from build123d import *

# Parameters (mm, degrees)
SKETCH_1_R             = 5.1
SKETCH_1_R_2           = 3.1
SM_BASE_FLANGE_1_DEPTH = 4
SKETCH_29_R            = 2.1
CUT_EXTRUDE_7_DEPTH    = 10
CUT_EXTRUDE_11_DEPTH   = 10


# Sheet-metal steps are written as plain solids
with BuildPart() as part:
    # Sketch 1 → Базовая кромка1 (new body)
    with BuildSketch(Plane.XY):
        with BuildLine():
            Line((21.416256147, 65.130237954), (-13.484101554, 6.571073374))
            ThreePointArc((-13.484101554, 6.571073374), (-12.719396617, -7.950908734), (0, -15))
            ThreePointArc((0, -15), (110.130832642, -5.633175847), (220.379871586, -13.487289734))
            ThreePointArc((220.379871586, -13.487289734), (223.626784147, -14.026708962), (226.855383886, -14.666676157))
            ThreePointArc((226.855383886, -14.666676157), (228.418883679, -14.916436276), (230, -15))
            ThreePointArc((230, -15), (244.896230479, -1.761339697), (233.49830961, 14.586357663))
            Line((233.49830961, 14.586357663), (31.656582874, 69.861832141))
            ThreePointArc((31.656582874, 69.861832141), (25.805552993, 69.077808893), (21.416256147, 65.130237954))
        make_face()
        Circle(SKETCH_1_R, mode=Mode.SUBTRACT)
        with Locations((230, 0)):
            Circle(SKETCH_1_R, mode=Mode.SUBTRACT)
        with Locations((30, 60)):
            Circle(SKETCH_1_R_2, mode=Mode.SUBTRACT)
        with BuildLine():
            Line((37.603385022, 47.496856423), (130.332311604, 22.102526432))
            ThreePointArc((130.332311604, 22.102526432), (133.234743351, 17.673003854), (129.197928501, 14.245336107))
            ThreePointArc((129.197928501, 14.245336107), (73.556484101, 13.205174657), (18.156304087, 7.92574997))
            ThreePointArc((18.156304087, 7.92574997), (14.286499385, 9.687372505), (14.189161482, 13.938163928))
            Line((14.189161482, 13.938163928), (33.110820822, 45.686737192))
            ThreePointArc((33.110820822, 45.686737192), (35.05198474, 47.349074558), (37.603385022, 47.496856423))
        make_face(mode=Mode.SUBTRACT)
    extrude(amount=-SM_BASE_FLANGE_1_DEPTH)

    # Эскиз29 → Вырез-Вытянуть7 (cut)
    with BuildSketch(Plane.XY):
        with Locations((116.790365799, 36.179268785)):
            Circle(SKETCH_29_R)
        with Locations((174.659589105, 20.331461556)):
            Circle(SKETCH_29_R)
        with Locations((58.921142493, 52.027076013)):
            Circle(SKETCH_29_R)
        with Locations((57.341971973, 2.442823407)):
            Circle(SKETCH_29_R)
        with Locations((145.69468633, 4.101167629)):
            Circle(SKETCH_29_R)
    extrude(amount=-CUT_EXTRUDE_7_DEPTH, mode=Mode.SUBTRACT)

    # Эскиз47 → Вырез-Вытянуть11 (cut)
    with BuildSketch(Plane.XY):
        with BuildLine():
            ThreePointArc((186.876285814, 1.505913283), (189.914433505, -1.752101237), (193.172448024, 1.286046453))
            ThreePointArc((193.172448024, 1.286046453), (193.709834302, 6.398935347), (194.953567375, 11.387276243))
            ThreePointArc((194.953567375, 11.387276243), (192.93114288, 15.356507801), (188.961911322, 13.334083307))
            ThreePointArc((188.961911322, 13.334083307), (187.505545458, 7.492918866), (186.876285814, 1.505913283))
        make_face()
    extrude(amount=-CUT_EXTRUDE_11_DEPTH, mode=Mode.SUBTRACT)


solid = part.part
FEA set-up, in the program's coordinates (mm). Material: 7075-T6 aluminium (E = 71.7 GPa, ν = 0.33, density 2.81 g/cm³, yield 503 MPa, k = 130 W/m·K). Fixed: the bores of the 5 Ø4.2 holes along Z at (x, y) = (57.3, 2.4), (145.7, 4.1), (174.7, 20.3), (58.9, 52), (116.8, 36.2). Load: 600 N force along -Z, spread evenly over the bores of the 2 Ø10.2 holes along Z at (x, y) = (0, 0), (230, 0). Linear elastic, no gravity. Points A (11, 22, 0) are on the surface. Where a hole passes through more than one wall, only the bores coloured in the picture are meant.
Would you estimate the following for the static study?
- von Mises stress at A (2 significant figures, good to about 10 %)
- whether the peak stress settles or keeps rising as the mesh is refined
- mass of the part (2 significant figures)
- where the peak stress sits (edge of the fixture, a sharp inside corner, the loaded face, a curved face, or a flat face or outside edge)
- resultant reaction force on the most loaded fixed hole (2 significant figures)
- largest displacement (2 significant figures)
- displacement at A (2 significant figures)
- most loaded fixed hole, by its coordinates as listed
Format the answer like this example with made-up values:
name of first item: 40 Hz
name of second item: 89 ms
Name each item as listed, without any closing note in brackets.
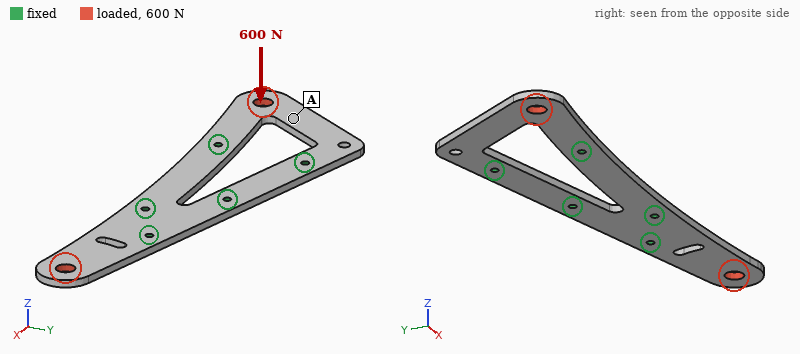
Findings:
von Mises stress at A: 52 MPa
whether the peak stress settles or keeps rising as the mesh is refined: keeps rising
mass of the part: 110 g
where the peak stress sits: edge of the fixture
resultant reaction force on the most loaded fixed hole: 530 N
largest displacement: 2.8 mm
displacement at A: 0.96 mm
most loaded fixed hole, by its coordinates as listed: (174.7, 20.3)
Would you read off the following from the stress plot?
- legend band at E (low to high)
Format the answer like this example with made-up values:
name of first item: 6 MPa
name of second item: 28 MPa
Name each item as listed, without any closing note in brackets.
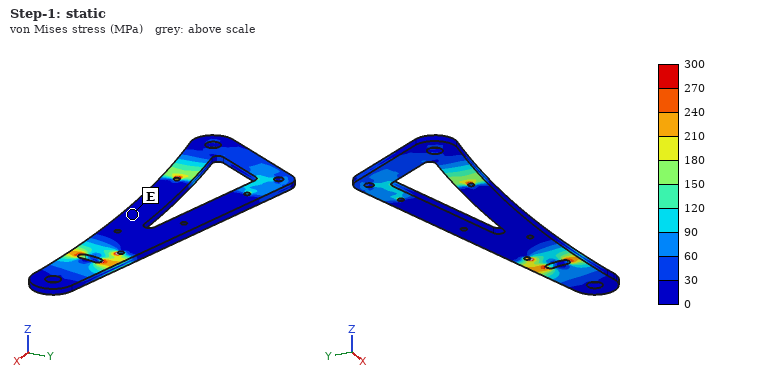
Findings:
legend band at E: 0 to 30 MPa
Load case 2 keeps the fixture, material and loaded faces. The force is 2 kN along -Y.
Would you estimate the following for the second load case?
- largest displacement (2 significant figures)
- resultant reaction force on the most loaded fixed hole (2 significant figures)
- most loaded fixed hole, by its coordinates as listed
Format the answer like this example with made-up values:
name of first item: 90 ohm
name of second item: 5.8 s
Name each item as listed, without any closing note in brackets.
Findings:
largest displacement: 0.15 mm
resultant reaction force on the most loaded fixed hole: 2.3 kN
most loaded fixed hole, by its coordinates as listed: (174.7, 20.3)
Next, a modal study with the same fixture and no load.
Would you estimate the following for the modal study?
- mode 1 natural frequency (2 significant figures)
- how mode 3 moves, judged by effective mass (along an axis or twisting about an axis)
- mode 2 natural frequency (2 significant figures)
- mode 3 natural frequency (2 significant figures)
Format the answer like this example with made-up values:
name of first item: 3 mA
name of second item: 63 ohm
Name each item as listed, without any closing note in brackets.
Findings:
mode 1 natural frequency: 630 Hz
how mode 3 moves, judged by effective mass: twisting about X
mode 2 natural frequency: 630 Hz
mode 3 natural frequency: 1700 Hz
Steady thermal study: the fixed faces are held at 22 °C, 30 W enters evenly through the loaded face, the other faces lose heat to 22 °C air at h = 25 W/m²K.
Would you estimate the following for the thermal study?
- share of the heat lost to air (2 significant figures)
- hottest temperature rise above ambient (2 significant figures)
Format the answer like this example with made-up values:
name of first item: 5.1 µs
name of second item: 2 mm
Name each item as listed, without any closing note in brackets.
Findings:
share of the heat lost to air: 27 %
hottest temperature rise above ambient: 57 K
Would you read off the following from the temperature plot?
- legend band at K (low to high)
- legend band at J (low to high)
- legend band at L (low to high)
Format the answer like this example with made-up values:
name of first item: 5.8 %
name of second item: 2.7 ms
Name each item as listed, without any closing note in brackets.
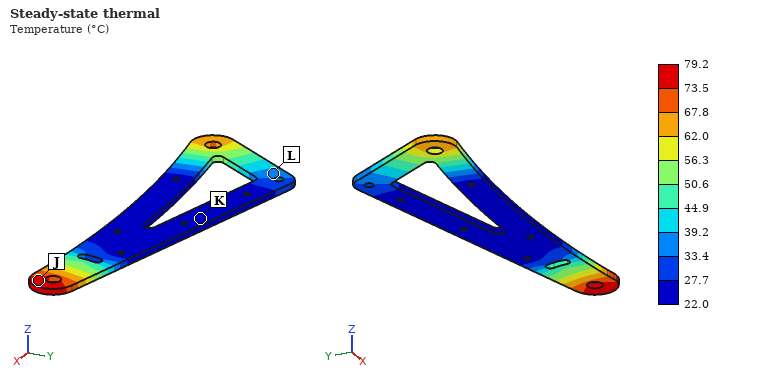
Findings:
legend band at K: 22.0 to 27.7 °C
legend band at J: 73.5 to 79.2 °C
legend band at L: 33.4 to 39.2 °C
